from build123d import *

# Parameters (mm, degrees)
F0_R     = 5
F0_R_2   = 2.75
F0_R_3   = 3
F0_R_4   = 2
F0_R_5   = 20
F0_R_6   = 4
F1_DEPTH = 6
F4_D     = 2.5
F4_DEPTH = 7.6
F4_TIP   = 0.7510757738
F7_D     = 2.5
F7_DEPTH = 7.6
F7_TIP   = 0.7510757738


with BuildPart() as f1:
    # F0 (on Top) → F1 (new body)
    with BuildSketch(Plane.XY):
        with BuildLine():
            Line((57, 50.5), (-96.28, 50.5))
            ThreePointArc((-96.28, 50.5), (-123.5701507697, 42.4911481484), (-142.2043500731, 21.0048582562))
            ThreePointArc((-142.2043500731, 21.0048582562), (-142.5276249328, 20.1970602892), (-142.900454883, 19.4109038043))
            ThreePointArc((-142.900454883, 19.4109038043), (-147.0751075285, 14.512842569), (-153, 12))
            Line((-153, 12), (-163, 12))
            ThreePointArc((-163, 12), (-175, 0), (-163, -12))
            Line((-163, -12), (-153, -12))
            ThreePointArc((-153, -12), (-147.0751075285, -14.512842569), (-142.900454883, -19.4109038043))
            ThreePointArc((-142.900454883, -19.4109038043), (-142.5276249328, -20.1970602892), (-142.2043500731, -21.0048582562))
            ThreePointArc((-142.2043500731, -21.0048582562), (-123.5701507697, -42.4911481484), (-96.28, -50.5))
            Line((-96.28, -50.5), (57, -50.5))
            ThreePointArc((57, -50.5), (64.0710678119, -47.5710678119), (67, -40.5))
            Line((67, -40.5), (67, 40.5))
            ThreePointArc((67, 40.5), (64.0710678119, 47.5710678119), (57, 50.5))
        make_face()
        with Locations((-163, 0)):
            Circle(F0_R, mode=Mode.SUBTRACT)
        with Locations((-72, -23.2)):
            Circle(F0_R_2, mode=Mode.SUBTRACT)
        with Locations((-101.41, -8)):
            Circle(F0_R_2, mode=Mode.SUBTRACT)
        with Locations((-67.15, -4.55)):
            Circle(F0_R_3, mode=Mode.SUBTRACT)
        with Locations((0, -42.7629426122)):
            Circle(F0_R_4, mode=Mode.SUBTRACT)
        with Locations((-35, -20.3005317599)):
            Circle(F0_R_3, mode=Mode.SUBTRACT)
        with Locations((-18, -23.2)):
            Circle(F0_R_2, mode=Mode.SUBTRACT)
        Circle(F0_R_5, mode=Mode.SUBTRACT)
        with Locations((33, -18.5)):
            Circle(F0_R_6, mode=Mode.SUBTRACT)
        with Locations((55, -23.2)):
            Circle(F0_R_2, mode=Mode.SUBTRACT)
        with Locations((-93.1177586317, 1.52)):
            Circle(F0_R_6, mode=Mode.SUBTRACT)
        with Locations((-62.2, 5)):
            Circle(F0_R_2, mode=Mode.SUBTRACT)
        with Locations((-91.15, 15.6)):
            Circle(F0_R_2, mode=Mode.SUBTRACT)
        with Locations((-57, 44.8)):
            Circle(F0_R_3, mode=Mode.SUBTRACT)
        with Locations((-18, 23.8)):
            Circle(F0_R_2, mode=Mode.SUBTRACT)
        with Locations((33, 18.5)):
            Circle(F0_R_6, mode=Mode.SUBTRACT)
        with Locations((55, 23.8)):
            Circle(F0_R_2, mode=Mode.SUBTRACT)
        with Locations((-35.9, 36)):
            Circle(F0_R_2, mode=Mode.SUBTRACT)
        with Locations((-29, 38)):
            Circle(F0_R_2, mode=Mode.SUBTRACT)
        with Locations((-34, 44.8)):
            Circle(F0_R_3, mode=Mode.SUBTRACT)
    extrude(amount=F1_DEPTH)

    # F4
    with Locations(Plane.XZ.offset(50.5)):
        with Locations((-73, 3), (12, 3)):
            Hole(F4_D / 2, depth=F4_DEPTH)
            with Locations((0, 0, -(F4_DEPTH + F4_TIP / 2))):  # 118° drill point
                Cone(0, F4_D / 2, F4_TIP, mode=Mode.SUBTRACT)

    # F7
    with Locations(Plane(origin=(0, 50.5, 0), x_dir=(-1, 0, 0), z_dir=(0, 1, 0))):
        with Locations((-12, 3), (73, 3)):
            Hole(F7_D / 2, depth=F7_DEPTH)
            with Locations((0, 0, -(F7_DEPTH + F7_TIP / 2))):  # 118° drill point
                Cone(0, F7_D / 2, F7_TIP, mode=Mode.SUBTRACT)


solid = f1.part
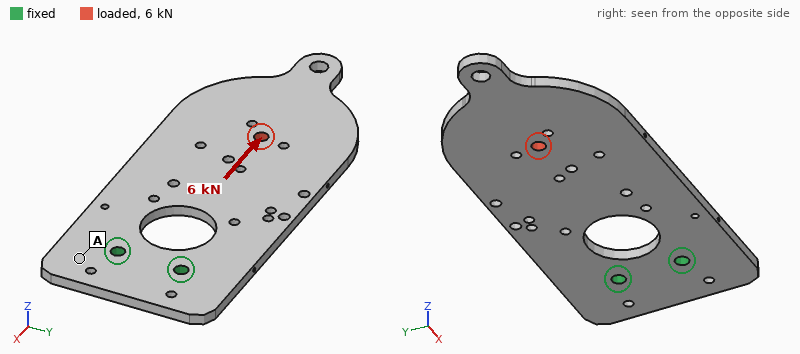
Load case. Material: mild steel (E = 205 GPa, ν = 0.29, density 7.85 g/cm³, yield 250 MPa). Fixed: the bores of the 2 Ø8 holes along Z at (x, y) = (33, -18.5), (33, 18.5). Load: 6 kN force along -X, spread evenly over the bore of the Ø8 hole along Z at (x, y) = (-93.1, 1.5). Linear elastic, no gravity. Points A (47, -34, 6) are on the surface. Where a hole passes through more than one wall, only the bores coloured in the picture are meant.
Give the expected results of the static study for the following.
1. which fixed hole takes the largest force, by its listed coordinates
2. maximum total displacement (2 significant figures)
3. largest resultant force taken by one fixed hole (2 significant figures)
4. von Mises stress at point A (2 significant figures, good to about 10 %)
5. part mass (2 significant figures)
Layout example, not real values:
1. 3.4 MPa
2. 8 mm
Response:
1. (33, 18.5)
2. 14 µm
3. 3.2 kN
4. 7.6 MPa
5. 910 g
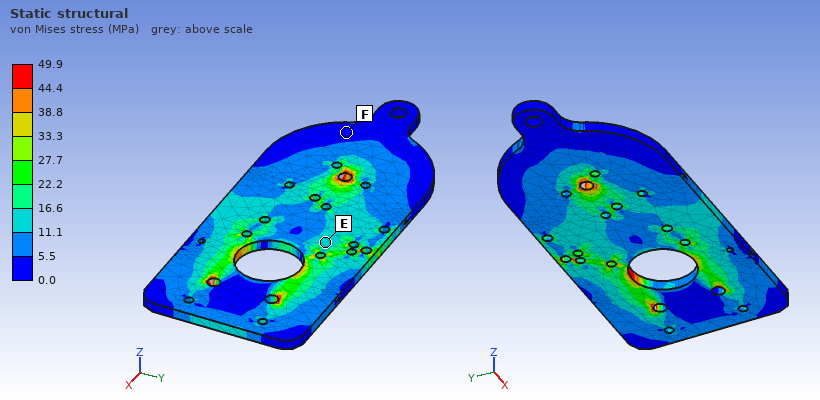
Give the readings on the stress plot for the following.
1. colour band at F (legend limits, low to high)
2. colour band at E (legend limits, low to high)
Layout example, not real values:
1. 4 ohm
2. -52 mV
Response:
1. 0.0 to 5.5 MPa
2. 11.1 to 16.6 MPa
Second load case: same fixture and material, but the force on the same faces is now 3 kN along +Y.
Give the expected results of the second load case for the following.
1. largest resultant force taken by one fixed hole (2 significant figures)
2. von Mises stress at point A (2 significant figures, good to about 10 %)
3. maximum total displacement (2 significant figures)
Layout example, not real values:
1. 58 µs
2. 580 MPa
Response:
1. 8.6 kN
2. 22 MPa
3. 0.12 mm
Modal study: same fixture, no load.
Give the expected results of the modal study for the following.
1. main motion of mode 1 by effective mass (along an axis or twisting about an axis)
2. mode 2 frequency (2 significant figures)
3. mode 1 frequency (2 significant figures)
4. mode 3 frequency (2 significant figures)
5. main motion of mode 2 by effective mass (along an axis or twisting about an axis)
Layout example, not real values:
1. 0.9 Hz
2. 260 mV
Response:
1. along Z
2. 590 Hz
3. 130 Hz
4. 840 Hz
5. twisting about X
